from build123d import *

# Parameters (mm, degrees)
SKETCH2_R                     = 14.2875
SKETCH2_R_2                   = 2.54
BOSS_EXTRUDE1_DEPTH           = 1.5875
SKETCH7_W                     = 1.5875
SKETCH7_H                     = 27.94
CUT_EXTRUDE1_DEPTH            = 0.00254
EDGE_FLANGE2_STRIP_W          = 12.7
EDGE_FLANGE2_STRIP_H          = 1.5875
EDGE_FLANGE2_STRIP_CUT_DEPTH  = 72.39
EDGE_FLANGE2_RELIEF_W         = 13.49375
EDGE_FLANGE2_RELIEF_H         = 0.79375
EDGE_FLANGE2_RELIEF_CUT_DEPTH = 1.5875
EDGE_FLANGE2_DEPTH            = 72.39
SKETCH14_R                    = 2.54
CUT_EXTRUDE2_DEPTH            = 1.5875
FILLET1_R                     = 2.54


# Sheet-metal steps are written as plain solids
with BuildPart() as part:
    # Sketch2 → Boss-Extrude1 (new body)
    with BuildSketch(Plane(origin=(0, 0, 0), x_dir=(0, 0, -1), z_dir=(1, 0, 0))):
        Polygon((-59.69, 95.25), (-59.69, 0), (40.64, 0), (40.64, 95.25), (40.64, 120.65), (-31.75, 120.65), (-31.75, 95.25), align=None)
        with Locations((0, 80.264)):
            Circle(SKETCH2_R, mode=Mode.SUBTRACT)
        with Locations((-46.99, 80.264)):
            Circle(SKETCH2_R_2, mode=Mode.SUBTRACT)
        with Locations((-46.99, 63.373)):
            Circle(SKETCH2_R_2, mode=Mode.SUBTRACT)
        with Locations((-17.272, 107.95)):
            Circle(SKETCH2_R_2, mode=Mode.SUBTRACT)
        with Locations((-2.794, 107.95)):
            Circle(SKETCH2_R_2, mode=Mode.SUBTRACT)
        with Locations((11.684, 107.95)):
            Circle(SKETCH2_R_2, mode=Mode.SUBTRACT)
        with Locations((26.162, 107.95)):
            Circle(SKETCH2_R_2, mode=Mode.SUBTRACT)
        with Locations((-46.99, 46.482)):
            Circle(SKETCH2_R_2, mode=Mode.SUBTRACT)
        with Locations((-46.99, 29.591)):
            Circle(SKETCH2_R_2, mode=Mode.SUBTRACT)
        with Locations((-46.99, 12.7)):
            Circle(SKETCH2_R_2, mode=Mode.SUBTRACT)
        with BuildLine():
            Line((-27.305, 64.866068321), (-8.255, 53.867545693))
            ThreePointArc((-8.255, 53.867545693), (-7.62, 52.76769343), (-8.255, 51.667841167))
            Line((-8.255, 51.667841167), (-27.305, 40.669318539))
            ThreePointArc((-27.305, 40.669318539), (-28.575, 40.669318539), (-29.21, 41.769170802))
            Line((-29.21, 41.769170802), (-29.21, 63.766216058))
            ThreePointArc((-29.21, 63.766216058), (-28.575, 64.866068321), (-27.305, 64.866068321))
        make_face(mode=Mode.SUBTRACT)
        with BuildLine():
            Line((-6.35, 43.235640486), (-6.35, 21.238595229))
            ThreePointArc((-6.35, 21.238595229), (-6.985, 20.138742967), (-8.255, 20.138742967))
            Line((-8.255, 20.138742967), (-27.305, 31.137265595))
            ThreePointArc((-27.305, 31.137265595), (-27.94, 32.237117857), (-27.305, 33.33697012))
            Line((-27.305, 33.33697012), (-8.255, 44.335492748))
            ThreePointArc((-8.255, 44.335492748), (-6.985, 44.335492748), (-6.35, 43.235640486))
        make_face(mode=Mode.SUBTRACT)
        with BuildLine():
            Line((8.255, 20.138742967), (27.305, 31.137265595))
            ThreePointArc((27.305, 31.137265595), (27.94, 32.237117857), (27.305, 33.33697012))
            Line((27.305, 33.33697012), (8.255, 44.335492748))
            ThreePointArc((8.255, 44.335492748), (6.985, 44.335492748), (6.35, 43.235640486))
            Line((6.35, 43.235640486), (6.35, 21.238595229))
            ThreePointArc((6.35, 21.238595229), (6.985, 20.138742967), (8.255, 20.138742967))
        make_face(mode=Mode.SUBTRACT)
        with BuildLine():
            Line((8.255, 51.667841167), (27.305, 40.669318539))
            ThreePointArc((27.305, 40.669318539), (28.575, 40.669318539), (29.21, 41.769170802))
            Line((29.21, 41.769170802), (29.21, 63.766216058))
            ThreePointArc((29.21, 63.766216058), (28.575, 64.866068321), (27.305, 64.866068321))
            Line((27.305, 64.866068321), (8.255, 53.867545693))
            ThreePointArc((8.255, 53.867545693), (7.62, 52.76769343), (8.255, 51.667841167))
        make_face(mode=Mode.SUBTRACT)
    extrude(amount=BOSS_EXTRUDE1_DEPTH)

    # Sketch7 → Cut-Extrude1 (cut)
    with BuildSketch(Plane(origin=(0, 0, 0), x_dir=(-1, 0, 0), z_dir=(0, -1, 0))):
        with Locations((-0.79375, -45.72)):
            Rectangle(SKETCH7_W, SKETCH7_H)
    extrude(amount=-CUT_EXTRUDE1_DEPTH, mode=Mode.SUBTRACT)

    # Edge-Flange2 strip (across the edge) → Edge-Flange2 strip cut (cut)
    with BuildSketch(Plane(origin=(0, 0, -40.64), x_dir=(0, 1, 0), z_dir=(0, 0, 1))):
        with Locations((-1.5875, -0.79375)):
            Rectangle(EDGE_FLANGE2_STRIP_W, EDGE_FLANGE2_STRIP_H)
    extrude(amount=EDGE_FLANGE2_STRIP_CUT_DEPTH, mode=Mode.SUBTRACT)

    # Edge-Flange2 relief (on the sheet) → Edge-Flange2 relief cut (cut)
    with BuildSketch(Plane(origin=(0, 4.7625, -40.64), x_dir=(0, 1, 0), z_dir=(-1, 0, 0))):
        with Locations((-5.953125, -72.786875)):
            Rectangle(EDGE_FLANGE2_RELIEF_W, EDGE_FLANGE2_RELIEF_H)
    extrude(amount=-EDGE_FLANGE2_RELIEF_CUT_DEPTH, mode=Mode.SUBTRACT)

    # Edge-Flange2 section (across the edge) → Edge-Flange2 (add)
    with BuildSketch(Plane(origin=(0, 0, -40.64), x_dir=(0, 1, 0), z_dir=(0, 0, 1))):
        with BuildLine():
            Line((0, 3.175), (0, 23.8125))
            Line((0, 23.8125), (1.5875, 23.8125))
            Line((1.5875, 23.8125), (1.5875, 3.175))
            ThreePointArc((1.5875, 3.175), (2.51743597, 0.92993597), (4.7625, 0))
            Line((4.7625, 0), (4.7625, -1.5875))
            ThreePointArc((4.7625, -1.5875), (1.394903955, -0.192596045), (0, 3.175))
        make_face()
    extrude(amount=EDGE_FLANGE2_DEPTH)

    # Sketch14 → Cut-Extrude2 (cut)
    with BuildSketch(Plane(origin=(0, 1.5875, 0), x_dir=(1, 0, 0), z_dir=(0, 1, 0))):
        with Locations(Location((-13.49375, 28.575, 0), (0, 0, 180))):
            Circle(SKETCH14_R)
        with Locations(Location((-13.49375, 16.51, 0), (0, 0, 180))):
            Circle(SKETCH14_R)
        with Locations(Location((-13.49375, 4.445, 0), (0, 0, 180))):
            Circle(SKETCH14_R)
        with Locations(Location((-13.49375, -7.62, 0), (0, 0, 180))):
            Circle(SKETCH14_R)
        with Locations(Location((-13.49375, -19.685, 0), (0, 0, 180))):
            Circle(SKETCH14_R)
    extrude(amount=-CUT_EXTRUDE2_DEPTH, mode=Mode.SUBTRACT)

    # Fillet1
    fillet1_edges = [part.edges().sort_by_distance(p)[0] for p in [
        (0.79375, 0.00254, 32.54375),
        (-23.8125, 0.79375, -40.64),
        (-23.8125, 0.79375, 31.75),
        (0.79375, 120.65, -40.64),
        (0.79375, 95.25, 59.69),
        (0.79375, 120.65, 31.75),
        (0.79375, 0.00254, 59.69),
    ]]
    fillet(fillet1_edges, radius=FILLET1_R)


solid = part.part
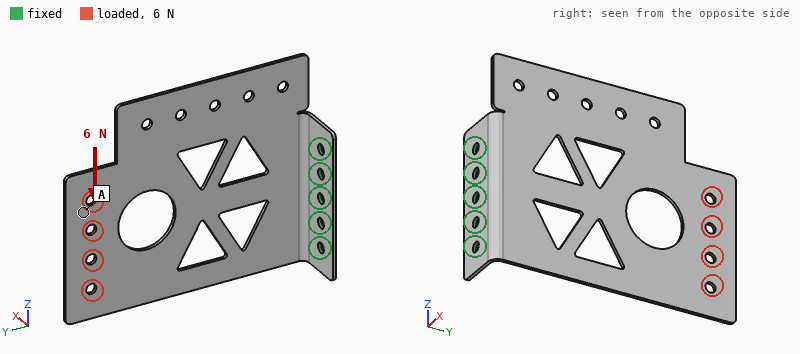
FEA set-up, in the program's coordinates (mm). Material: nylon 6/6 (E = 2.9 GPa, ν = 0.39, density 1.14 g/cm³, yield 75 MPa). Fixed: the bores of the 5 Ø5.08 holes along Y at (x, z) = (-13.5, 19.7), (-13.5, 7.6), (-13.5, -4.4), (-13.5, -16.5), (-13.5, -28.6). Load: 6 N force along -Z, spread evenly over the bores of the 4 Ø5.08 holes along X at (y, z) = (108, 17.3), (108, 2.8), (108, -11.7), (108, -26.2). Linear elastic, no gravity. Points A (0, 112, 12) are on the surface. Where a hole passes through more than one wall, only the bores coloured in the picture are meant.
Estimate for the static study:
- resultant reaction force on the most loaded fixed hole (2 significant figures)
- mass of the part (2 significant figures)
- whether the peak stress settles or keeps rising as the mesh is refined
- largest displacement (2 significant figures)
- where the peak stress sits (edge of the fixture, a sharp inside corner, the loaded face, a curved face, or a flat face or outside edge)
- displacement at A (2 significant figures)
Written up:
11 N
20 g
keeps rising
1.8 mm
edge of the fixture
1.3 mm
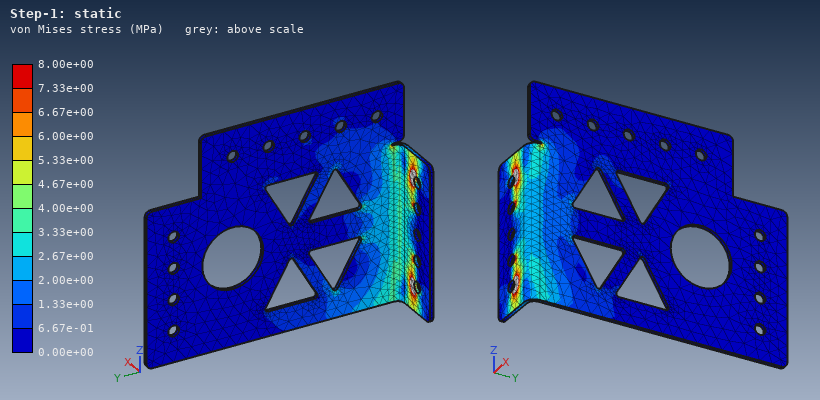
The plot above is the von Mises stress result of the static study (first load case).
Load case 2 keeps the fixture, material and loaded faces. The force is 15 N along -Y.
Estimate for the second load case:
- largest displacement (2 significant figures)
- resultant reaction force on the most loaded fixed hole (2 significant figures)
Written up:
1.9 mm
3.4 N
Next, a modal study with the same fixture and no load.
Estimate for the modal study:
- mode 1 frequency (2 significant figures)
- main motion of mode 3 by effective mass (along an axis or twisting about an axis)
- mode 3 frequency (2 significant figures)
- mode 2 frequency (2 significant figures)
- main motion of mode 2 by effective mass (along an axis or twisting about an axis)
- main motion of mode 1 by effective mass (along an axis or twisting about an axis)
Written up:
24 Hz
along Z
140 Hz
66 Hz
twisting about Y
along X
